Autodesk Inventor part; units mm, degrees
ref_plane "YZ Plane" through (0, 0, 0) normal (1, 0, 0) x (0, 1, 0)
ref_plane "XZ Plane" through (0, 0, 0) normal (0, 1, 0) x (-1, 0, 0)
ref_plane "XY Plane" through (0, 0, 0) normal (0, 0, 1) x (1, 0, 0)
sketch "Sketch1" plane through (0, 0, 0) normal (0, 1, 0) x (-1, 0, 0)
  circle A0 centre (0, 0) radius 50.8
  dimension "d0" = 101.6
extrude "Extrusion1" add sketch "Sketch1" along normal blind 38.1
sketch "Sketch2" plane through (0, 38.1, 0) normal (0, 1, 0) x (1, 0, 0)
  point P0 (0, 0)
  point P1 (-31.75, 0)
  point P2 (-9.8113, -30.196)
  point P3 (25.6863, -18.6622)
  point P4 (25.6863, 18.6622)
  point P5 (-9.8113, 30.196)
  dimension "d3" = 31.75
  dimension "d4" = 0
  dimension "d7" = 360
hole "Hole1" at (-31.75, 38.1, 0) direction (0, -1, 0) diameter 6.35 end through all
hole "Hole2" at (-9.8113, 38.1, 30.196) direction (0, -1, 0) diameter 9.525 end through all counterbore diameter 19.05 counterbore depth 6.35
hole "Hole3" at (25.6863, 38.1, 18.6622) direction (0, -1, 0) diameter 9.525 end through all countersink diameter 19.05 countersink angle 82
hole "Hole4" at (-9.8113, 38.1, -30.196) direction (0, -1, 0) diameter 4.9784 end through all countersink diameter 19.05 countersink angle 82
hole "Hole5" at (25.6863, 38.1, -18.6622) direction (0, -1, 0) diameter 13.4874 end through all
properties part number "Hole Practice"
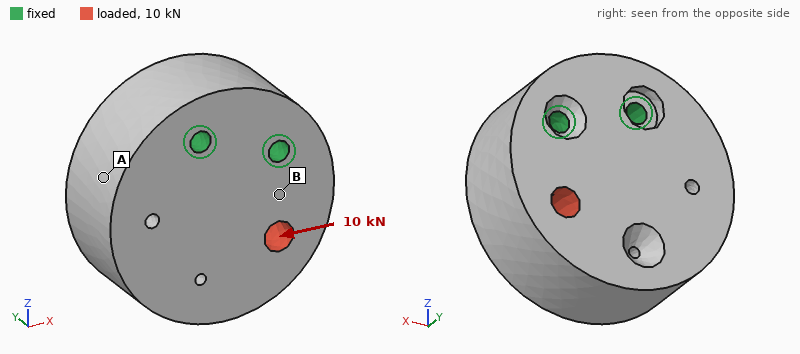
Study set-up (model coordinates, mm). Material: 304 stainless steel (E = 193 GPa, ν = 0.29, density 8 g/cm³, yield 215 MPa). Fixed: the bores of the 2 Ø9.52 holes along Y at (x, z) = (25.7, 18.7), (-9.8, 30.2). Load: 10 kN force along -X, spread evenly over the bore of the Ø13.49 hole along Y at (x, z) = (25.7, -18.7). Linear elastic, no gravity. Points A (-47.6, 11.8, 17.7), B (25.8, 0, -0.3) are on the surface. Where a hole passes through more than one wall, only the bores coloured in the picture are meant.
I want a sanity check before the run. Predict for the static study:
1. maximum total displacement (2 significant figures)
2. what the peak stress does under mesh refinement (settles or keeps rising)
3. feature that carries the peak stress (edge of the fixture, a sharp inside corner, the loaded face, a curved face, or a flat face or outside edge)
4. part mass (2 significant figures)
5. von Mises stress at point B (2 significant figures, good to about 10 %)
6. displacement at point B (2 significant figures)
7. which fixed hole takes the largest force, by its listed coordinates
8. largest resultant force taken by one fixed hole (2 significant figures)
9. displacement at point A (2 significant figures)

6.0 µm
keeps rising
edge of the fixture
2.3 kg
9.3 MPa
2.2 µm
(25.7, 18.7)
12 kN
3.4 µm
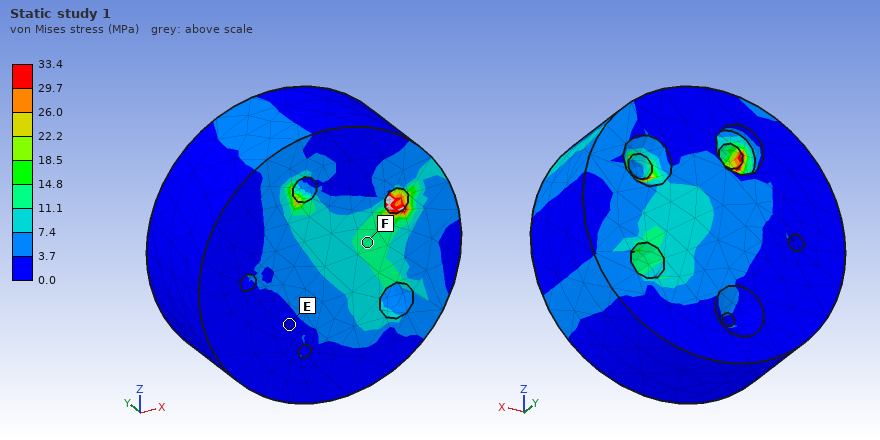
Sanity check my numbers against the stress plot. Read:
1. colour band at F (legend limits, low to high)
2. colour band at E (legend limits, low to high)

11.1 to 14.8 MPa
0.0 to 3.7 MPa
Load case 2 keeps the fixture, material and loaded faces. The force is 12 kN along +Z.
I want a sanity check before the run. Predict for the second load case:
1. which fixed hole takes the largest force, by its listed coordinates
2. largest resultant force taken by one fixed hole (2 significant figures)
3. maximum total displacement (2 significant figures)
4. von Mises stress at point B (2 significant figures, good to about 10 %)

(25.7, 18.7)
11 kN
2.9 µm
10 MPa
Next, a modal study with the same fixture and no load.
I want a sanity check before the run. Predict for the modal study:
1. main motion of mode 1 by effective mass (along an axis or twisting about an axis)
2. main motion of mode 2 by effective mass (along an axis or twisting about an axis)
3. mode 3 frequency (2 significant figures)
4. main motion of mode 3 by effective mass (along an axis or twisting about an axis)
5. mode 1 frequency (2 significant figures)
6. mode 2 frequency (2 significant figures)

along Y
along X
7800 Hz
twisting about Z
4200 Hz
5800 Hz
